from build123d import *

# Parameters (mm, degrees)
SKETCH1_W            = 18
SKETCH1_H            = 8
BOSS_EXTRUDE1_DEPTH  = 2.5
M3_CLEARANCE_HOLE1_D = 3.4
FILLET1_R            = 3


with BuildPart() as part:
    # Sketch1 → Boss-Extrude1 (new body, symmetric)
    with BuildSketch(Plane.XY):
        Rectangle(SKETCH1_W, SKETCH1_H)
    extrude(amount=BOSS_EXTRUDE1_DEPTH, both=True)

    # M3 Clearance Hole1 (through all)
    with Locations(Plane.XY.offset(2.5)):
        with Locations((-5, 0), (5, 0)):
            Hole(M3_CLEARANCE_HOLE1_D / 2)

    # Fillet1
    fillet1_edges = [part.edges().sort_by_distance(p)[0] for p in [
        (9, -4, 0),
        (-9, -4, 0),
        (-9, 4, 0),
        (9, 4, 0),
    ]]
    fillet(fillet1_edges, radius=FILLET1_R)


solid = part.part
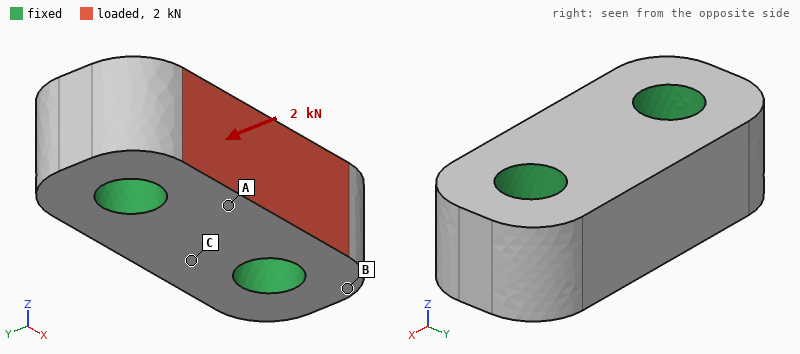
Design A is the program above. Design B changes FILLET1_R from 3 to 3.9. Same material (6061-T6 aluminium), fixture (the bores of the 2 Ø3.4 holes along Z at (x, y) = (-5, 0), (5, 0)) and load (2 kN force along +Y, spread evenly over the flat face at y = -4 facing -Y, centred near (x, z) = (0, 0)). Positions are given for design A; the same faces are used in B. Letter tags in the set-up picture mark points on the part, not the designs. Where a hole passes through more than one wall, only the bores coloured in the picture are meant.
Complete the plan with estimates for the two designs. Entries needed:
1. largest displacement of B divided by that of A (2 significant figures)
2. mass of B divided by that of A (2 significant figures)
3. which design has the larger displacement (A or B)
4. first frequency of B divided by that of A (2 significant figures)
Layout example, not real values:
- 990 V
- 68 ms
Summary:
- 1.2
- 0.95
- B
- 1.0
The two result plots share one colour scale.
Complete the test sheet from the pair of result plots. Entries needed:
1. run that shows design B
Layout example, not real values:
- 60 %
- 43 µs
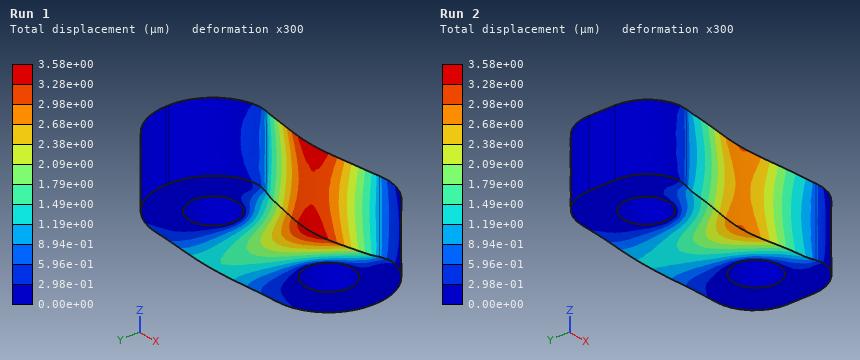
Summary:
- Run 1
